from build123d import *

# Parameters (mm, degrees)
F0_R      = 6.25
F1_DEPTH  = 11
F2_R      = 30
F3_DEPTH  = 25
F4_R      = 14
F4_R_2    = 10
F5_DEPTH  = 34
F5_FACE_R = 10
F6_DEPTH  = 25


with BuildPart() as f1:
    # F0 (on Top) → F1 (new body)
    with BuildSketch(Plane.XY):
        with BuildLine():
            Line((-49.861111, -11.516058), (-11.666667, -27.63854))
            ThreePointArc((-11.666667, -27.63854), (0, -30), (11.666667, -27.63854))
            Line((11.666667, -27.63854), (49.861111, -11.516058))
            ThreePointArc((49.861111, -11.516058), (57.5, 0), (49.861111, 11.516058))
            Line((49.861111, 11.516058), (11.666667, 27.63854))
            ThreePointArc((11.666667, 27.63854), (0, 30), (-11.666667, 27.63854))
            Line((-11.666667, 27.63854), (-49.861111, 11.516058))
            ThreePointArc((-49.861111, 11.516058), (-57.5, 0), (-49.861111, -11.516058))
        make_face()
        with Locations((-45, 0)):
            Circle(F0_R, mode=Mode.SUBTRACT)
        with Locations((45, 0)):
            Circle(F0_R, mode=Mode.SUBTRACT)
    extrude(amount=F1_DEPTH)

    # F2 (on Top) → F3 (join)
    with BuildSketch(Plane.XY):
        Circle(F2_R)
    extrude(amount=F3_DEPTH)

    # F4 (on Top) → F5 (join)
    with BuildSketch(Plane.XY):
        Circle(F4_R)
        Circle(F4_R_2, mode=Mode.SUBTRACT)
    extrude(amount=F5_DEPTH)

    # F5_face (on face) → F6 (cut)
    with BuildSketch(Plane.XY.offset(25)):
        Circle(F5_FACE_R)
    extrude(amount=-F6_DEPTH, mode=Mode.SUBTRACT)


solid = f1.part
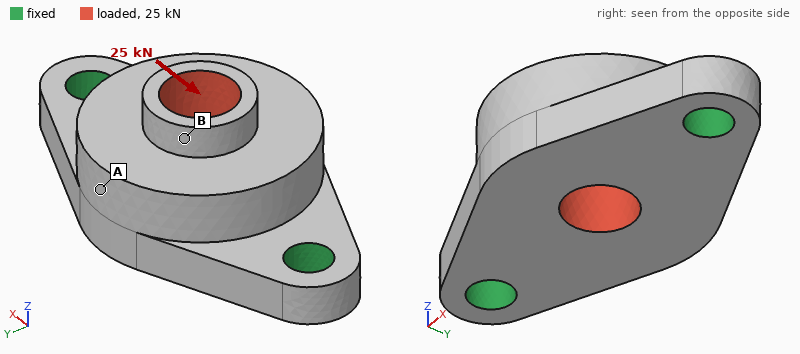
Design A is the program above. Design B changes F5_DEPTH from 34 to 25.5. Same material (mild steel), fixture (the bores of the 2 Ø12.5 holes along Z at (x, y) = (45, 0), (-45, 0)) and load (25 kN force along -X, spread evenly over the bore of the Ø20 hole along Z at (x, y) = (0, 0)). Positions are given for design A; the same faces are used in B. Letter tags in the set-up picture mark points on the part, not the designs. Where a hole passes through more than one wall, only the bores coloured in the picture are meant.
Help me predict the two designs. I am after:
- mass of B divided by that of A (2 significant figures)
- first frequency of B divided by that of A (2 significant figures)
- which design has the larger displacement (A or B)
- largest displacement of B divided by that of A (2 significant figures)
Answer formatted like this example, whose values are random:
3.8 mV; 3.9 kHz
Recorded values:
0.97; 1.0; A; 0.50
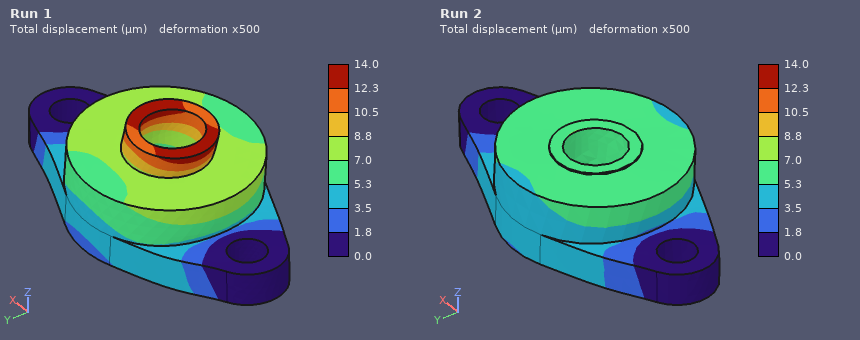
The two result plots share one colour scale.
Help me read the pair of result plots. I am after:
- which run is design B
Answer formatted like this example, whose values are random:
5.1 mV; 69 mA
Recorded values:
Run 2
